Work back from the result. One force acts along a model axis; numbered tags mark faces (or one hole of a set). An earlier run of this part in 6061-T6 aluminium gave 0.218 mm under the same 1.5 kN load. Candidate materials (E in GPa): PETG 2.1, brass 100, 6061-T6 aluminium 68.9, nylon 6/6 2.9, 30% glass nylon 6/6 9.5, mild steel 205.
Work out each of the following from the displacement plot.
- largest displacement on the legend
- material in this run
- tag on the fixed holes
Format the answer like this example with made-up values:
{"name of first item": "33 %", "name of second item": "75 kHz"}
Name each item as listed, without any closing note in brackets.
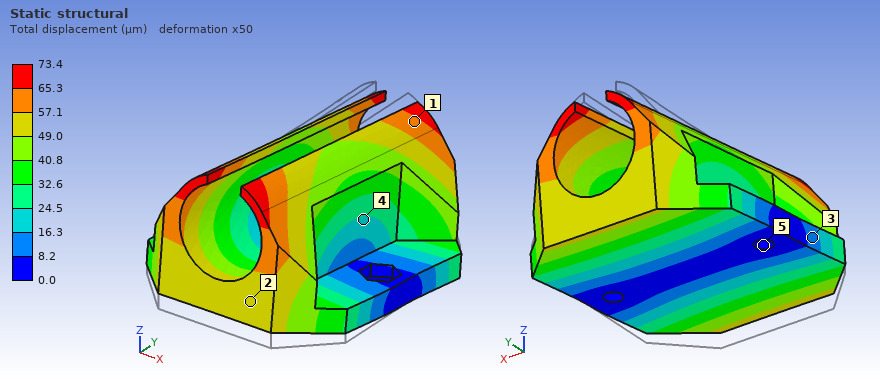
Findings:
{"largest displacement on the legend": "73.4 µm", "material in this run": "mild steel", "tag on the fixed holes": "5"}
